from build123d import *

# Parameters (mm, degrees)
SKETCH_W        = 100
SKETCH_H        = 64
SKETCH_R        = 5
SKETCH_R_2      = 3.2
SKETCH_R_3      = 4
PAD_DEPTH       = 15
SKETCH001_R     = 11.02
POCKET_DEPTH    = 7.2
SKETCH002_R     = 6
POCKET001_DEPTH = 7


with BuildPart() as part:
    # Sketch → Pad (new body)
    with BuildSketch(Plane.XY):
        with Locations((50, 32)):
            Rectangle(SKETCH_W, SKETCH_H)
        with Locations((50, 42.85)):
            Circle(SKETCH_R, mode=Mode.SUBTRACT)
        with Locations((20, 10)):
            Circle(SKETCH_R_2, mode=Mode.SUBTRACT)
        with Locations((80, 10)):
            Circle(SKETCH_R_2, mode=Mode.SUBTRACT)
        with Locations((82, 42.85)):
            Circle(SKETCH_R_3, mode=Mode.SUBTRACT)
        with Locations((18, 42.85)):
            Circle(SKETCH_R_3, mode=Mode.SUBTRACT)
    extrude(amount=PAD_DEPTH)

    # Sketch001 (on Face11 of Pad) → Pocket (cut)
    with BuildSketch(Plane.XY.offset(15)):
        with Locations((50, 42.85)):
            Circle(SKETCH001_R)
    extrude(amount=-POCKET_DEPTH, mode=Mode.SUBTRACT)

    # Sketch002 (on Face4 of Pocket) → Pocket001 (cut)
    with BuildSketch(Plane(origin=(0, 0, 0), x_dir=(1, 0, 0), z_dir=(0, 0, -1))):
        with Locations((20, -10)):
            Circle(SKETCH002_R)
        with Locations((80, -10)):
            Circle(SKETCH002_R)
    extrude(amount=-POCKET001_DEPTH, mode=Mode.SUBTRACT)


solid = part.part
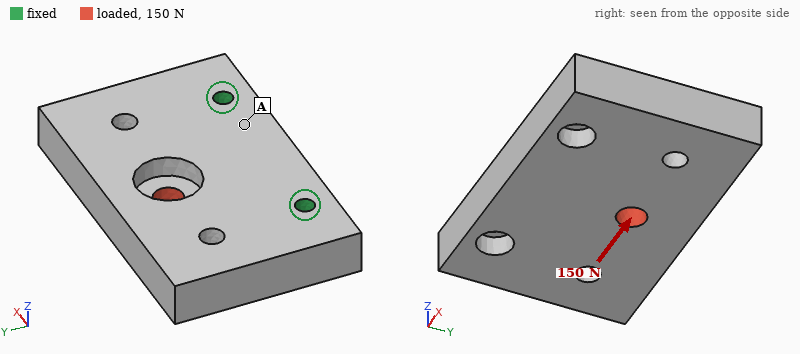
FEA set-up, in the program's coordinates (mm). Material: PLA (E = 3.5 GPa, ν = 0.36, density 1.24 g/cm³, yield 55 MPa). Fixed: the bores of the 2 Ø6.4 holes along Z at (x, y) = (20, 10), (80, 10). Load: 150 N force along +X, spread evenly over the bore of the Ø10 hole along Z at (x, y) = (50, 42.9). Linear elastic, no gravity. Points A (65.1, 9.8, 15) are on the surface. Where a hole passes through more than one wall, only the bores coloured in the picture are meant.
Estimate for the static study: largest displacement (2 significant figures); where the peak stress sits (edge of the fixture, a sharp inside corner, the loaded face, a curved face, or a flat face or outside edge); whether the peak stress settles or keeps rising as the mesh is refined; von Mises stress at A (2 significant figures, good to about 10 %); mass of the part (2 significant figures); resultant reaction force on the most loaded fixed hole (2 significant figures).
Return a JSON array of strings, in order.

["9.5 µm", "edge of the fixture", "keeps rising", "0.24 MPa", "110 g", "110 N"]
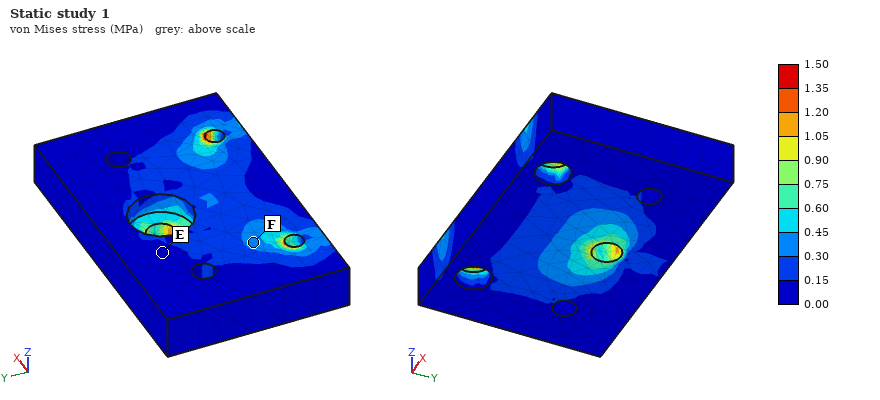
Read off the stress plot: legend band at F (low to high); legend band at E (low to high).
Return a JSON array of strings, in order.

["0.30 to 0.45 MPa", "0.00 to 0.15 MPa"]
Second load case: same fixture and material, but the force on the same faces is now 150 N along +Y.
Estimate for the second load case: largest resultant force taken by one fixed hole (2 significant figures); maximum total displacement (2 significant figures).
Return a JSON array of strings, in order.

["78 N", "35 µm"]
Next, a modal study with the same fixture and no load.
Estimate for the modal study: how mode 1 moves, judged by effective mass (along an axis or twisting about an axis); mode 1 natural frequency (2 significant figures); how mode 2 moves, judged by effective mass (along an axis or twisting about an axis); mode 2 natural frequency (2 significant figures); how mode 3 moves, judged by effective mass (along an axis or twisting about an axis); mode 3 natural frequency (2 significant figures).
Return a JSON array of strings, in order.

["along Z", "700 Hz", "twisting about Y", "1400 Hz", "along X", "2600 Hz"]
